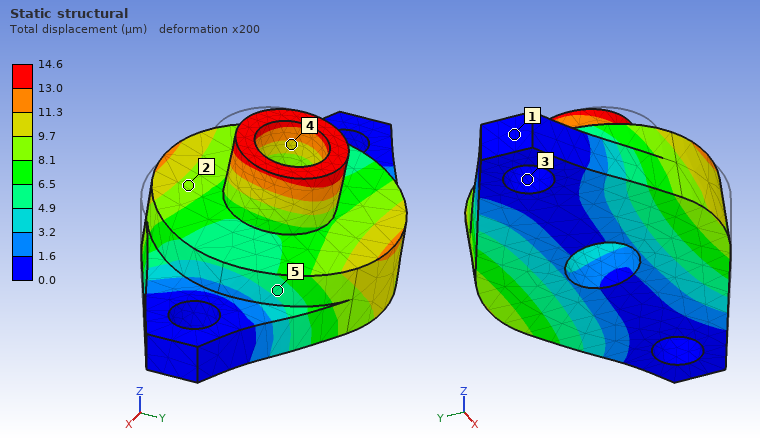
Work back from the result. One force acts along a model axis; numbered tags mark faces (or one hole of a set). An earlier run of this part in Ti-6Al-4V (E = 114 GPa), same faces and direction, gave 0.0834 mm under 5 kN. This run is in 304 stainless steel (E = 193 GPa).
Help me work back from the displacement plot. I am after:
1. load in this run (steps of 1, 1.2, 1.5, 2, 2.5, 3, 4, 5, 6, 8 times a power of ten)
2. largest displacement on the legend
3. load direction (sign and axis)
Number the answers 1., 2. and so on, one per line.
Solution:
1. 1.5 kN
2. 14.6 µm
3. +Y
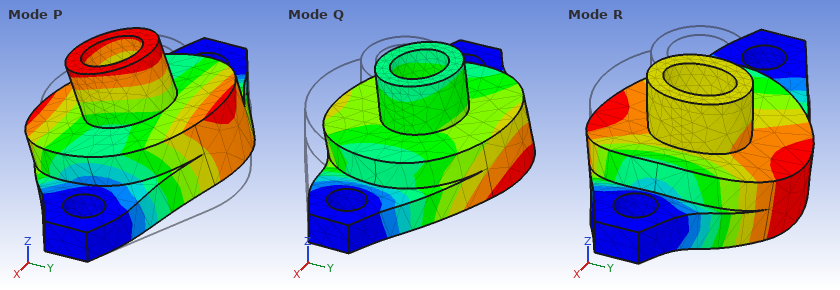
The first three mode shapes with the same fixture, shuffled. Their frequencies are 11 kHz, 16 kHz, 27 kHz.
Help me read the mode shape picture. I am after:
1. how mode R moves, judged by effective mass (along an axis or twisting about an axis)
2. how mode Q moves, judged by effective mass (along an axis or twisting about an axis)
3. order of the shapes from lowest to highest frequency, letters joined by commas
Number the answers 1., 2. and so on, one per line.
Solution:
1. along Z
2. along Y
3. P, R, Q
